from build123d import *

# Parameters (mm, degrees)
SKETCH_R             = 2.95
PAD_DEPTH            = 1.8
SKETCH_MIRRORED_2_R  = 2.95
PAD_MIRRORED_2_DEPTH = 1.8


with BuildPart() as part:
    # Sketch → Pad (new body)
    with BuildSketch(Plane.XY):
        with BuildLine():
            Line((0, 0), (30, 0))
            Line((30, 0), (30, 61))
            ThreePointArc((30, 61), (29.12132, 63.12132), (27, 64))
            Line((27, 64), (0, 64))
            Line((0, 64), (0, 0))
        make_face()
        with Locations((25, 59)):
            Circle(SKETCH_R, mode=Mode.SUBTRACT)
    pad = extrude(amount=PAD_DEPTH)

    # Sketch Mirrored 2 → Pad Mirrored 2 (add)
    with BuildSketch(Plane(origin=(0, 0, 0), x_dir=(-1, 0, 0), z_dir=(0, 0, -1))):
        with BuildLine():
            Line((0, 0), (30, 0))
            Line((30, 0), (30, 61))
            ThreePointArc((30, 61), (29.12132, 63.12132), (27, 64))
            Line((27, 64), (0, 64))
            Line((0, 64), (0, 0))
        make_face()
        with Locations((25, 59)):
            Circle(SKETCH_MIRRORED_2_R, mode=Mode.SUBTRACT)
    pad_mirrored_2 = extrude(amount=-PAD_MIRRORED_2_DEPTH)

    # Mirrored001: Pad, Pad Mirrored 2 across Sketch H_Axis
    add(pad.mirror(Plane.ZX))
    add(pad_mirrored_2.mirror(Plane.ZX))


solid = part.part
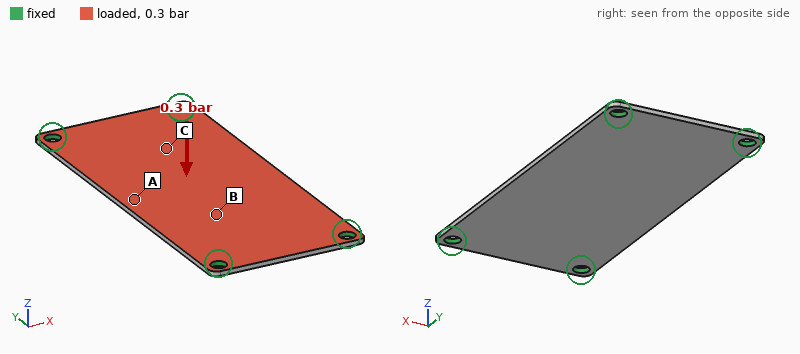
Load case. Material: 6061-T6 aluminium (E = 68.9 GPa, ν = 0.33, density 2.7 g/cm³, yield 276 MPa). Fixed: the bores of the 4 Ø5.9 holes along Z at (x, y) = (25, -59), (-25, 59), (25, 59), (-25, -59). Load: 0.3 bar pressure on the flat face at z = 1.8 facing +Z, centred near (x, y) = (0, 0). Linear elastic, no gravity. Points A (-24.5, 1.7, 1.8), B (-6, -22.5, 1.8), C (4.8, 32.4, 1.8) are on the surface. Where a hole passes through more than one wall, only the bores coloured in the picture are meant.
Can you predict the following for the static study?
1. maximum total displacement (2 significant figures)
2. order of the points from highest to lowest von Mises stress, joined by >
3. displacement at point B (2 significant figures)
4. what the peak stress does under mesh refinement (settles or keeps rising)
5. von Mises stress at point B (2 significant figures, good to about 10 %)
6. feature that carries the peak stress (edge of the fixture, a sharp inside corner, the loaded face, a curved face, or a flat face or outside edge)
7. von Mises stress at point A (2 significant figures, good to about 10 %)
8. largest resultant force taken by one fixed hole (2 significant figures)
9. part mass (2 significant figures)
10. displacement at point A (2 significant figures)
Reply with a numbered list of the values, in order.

1. 0.50 mm
2. A > B > C
3. 0.36 mm
4. keeps rising
5. 17 MPa
6. edge of the fixture
7. 34 MPa
8. 57 N
9. 37 g
10. 0.48 mm
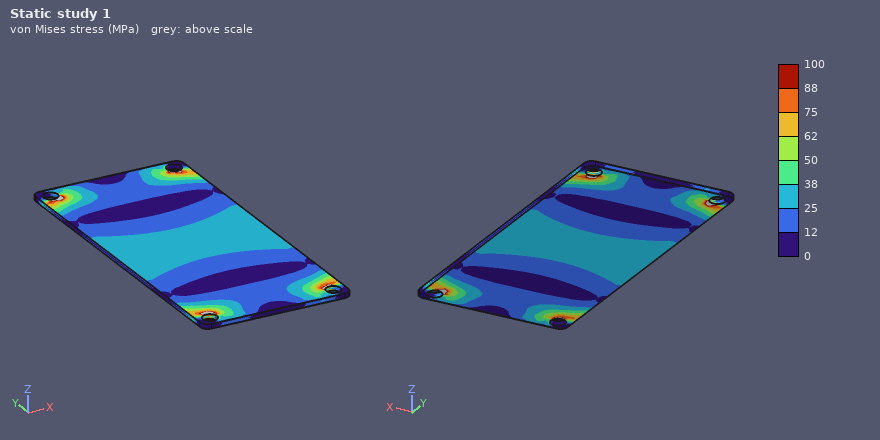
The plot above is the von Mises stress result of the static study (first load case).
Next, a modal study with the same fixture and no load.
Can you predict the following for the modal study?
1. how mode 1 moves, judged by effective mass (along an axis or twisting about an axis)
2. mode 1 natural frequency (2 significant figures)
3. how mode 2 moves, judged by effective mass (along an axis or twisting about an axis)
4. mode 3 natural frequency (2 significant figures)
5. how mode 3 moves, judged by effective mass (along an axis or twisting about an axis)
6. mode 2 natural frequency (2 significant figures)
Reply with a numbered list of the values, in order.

1. along Z
2. 650 Hz
3. twisting about Y
4. 1800 Hz
5. twisting about X
6. 1200 Hz
